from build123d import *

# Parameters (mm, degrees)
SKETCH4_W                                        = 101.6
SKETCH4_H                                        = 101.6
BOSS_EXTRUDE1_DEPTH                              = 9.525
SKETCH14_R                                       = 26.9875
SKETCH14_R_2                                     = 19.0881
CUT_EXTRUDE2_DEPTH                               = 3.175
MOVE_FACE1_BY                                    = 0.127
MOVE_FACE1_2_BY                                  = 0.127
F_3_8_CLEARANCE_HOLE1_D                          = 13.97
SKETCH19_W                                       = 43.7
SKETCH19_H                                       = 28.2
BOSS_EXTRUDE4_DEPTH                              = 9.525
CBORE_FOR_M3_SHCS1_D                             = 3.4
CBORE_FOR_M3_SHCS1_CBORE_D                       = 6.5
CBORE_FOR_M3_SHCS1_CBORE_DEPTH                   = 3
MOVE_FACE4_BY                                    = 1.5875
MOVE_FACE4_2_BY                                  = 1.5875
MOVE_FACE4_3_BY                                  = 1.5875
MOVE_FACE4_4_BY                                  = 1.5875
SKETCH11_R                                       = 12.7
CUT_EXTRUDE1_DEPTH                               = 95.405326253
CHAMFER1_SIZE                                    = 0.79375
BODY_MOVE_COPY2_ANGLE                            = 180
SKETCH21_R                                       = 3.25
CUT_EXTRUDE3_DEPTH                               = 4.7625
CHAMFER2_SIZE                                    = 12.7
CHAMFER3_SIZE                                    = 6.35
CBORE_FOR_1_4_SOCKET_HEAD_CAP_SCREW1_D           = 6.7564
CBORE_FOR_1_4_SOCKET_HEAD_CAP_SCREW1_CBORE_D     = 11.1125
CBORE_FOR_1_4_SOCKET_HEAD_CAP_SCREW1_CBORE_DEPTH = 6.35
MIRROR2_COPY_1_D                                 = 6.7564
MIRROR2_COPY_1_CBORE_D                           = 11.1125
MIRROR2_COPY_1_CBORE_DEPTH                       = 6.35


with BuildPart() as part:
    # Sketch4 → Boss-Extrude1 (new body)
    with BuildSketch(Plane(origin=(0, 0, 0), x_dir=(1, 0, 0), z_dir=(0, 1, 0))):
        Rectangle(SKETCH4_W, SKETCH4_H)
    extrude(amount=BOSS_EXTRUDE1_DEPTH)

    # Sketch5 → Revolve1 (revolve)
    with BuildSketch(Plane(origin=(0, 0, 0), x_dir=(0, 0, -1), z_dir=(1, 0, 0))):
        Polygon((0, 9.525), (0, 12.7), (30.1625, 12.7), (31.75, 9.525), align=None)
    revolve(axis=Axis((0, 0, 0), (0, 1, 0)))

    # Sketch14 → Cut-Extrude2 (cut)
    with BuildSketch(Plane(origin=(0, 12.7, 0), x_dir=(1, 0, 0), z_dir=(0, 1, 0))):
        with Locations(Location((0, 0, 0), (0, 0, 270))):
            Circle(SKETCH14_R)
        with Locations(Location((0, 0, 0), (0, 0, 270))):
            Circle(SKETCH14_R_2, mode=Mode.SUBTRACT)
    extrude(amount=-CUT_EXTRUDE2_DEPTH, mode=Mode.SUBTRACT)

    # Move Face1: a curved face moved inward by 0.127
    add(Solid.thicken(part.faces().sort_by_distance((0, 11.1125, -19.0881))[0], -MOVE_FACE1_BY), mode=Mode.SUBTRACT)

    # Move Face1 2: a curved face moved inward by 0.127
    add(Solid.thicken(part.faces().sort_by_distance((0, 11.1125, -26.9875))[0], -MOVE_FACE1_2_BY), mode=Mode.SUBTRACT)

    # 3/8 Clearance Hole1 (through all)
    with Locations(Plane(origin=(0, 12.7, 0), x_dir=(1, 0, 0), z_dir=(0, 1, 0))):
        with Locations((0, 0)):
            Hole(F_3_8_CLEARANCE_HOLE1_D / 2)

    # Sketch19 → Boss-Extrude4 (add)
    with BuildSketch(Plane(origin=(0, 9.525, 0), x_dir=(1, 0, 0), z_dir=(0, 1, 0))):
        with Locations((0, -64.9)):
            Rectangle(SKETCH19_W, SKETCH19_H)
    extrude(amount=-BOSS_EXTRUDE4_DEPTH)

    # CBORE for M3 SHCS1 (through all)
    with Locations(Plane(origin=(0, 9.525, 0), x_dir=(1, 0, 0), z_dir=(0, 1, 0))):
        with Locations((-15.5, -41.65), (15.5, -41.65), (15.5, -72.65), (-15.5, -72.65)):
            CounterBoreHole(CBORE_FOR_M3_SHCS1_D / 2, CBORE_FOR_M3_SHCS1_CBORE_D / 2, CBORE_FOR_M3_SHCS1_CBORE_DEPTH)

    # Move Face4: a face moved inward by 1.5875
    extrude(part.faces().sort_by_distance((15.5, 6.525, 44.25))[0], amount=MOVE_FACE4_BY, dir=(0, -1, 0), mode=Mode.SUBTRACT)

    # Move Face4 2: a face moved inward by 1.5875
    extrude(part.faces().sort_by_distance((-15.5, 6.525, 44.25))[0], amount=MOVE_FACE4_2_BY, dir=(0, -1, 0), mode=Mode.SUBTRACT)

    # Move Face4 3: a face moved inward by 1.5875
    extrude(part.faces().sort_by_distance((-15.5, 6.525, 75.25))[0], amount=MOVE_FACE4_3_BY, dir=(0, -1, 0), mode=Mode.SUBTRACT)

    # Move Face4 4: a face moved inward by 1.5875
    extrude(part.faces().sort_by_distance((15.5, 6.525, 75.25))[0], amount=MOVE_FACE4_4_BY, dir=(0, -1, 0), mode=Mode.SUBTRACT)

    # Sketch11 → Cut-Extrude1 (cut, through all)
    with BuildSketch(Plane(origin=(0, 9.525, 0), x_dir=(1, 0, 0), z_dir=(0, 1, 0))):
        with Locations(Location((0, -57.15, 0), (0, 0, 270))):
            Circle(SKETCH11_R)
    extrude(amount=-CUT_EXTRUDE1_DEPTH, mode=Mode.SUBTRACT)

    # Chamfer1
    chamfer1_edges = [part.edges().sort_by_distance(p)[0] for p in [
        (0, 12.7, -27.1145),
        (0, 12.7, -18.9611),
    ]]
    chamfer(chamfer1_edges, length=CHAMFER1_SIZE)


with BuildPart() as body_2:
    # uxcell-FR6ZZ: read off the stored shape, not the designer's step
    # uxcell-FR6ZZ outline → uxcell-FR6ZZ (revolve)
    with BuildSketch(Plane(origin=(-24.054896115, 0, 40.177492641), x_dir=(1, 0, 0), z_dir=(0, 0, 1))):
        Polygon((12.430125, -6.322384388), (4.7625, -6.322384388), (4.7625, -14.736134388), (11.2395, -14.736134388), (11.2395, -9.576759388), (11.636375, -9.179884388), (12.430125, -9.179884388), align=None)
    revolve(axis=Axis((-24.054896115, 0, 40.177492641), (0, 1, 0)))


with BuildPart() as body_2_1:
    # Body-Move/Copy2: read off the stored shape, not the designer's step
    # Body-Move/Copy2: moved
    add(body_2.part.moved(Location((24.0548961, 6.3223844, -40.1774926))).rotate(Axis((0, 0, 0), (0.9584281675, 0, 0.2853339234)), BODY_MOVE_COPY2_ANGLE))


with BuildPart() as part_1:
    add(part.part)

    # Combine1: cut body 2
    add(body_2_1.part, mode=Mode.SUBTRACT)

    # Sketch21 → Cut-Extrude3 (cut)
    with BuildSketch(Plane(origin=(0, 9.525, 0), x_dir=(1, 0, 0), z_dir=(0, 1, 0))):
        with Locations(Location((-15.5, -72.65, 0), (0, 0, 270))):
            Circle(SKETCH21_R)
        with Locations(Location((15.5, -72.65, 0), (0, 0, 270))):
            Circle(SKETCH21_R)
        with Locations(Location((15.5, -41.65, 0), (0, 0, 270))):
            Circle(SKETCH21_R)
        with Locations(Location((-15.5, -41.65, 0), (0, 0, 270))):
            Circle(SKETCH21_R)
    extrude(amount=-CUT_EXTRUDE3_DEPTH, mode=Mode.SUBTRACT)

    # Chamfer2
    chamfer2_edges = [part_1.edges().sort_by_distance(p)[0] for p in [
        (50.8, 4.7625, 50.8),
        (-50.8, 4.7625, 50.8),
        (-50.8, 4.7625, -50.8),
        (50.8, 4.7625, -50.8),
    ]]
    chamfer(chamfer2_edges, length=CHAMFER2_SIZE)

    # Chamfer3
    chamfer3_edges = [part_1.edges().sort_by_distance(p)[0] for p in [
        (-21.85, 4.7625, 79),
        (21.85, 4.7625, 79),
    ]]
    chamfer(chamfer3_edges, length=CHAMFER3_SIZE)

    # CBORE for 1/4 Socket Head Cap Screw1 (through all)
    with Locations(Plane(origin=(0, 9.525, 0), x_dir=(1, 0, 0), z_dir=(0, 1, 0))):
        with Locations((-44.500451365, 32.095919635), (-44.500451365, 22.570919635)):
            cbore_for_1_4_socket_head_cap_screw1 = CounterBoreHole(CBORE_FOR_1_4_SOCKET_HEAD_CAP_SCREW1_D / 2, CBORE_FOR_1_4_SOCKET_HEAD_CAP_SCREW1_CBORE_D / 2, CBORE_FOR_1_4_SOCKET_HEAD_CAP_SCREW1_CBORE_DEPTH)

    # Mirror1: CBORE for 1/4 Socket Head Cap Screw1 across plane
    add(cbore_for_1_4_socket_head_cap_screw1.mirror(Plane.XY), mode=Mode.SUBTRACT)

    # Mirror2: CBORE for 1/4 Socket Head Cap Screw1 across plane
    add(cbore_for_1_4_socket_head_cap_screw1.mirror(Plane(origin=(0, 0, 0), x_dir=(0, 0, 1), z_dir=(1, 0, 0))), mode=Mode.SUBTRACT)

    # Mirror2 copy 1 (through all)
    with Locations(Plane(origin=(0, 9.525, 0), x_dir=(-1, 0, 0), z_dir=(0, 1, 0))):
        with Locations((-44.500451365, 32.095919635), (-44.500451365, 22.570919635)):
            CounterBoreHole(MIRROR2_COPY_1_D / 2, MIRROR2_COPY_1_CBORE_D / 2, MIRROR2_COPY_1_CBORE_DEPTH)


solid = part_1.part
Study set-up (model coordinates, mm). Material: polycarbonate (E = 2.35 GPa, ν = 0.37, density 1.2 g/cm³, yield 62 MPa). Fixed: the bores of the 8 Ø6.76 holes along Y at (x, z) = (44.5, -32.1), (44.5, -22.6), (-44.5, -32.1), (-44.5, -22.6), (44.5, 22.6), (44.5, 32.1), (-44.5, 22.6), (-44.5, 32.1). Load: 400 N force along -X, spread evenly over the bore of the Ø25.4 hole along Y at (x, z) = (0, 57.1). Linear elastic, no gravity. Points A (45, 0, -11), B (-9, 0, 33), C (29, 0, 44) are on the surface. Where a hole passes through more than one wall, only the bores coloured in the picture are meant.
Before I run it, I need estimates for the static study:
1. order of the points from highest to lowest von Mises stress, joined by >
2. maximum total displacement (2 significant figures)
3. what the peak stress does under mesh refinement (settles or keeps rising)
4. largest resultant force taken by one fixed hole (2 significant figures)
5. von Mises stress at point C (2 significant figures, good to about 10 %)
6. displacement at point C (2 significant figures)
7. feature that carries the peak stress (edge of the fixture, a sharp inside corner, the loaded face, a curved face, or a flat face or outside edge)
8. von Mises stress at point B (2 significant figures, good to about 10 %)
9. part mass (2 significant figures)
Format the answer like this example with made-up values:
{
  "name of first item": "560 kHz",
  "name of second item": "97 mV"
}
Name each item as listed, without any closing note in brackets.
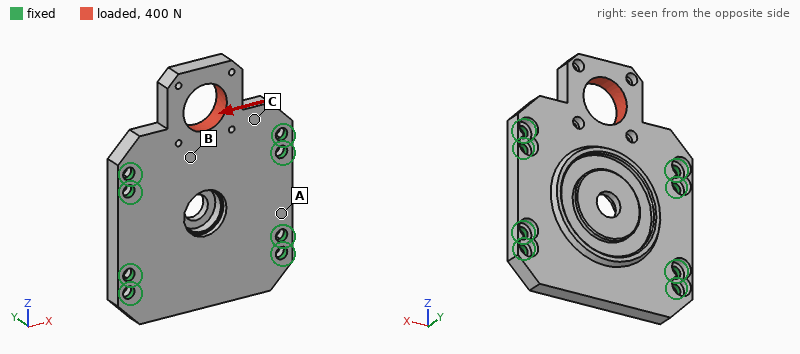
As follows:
{
  "order of the points from highest to lowest von Mises stress, joined by >": "C > B > A",
  "maximum total displacement": "0.12 mm",
  "what the peak stress does under mesh refinement": "keeps rising",
  "largest resultant force taken by one fixed hole": "130 N",
  "von Mises stress at point C": "2.0 MPa",
  "displacement at point C": "0.020 mm",
  "feature that carries the peak stress": "edge of the fixture",
  "von Mises stress at point B": "0.91 MPa",
  "part mass": "120 g"
}
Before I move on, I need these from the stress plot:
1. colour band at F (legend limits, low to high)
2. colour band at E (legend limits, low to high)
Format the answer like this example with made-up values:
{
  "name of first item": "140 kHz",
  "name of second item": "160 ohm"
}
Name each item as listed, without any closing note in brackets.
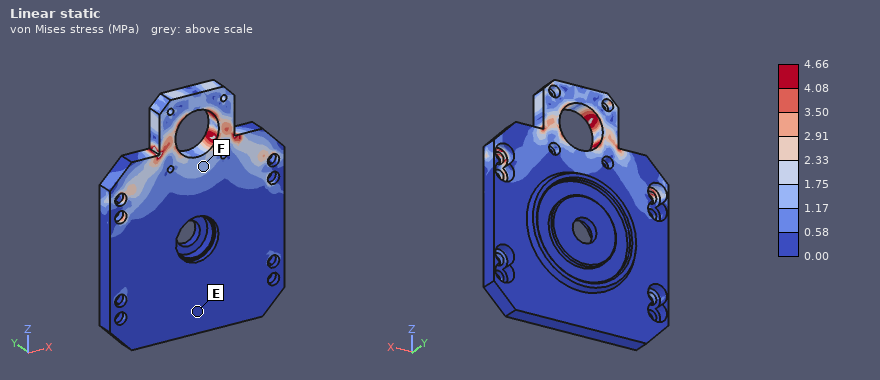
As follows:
{
  "colour band at F": "1.17 to 1.75 MPa",
  "colour band at E": "0.00 to 0.58 MPa"
}
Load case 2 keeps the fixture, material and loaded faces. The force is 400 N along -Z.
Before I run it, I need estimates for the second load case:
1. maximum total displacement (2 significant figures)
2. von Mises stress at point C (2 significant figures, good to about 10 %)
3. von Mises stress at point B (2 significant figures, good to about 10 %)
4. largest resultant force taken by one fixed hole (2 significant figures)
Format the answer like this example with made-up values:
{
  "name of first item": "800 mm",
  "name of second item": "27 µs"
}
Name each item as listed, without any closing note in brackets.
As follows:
{
  "maximum total displacement": "48 µm",
  "von Mises stress at point C": "0.77 MPa",
  "von Mises stress at point B": "0.52 MPa",
  "largest resultant force taken by one fixed hole": "71 N"
}
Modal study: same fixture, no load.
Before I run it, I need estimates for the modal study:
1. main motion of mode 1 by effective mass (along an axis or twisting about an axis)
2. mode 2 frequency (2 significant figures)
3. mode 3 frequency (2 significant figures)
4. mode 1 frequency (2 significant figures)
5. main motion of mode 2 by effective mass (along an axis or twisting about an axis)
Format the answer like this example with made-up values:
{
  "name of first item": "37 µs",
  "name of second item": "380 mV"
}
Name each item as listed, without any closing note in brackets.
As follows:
{
  "main motion of mode 1 by effective mass": "along Y",
  "mode 2 frequency": "1200 Hz",
  "mode 3 frequency": "1600 Hz",
  "mode 1 frequency": "700 Hz",
  "main motion of mode 2 by effective mass": "along Y"
}
